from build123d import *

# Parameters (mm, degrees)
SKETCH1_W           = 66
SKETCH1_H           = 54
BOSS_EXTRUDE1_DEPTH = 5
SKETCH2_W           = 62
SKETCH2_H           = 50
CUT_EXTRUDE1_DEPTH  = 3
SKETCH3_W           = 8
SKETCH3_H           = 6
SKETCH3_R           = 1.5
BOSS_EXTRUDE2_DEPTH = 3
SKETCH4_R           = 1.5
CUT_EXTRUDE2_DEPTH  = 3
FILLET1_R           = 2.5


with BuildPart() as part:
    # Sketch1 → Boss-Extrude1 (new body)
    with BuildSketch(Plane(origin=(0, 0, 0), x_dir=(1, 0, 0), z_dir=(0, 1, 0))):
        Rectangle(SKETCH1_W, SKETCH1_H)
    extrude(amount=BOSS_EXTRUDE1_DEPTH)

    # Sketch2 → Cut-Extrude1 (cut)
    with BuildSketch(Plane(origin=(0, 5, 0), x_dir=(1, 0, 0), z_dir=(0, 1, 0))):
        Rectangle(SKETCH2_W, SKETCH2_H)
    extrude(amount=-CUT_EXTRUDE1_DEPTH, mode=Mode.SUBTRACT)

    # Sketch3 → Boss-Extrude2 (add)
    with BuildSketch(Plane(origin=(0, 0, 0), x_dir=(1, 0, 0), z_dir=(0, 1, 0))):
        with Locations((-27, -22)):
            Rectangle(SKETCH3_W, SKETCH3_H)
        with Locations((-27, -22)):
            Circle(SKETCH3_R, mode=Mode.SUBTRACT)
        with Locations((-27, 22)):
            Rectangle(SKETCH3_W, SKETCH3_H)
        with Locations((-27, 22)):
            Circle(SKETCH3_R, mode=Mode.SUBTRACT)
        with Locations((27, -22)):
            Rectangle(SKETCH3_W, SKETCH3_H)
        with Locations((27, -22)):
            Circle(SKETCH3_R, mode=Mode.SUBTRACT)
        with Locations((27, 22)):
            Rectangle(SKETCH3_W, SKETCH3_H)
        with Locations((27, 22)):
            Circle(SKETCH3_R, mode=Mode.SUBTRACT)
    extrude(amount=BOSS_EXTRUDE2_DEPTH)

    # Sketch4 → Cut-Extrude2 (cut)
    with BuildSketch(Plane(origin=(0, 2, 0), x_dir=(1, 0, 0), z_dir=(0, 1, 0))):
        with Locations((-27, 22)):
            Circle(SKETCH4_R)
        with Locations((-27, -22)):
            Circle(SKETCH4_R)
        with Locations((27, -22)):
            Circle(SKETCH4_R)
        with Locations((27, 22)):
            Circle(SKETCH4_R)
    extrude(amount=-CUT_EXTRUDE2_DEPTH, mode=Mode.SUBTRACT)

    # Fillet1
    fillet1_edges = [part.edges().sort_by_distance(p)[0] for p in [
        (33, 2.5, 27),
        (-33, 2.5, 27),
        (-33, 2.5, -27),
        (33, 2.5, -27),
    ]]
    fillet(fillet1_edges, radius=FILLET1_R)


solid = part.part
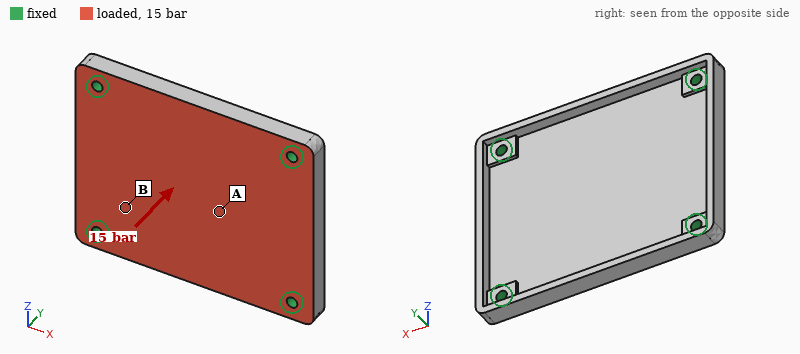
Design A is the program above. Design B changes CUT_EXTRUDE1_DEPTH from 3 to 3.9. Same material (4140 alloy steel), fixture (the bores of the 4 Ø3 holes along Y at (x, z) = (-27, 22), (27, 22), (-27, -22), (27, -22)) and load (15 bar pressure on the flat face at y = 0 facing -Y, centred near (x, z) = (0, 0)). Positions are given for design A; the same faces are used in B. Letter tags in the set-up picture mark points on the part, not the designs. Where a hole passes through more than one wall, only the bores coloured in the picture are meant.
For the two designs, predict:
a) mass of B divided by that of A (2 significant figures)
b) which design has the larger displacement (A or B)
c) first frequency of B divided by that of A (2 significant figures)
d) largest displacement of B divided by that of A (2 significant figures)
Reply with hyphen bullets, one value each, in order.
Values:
- 0.70
- B
- 0.69
- 3.9
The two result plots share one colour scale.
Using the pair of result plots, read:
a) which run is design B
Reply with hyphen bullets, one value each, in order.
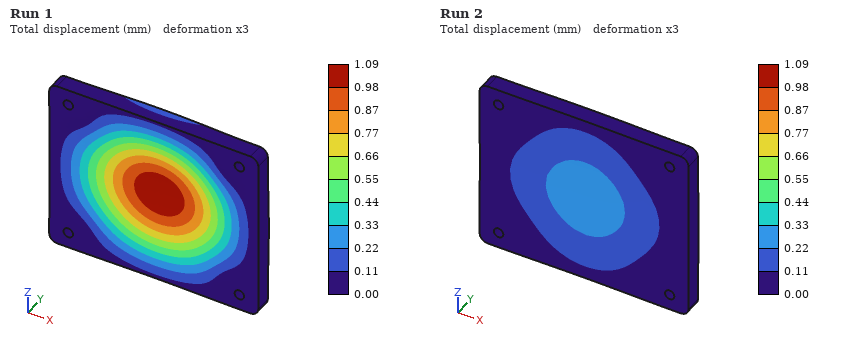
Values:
- Run 1
